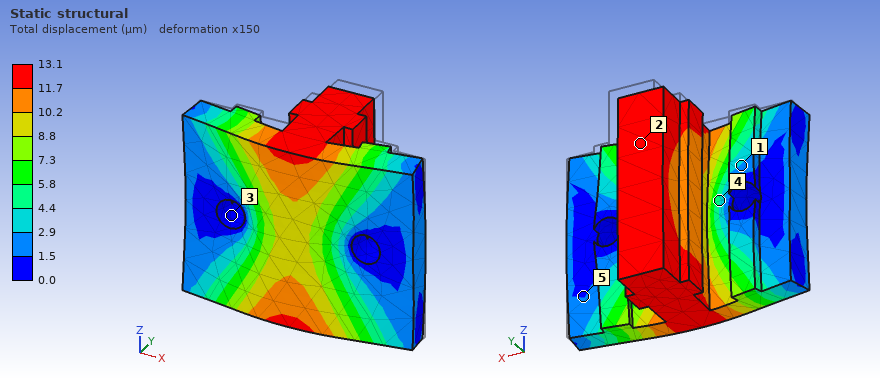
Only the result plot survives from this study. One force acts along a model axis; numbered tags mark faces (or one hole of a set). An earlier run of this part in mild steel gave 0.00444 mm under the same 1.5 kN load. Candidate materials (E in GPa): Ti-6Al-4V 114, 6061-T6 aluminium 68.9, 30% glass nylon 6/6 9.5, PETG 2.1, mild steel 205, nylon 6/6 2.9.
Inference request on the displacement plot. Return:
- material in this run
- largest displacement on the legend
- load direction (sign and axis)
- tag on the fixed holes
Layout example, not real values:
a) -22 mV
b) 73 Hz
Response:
a) 6061-T6 aluminium
b) 13.1 µm
c) -Y
d) 3
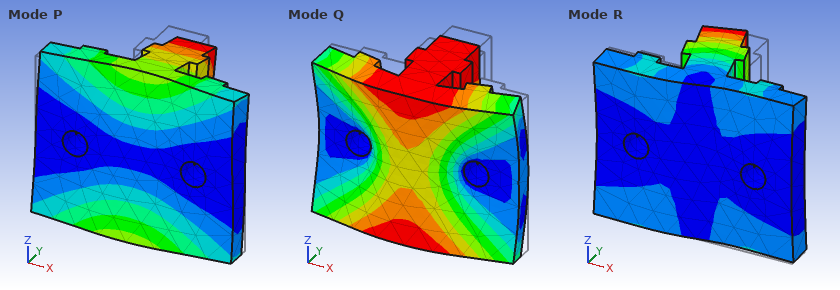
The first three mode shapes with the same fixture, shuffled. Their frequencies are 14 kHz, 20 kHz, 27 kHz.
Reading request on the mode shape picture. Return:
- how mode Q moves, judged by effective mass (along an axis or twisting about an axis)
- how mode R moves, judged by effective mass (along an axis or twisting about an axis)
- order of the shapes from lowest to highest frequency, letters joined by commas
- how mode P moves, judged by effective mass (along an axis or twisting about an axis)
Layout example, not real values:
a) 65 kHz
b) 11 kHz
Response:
a) along Y
b) along X
c) P, R, Q
d) along Z
